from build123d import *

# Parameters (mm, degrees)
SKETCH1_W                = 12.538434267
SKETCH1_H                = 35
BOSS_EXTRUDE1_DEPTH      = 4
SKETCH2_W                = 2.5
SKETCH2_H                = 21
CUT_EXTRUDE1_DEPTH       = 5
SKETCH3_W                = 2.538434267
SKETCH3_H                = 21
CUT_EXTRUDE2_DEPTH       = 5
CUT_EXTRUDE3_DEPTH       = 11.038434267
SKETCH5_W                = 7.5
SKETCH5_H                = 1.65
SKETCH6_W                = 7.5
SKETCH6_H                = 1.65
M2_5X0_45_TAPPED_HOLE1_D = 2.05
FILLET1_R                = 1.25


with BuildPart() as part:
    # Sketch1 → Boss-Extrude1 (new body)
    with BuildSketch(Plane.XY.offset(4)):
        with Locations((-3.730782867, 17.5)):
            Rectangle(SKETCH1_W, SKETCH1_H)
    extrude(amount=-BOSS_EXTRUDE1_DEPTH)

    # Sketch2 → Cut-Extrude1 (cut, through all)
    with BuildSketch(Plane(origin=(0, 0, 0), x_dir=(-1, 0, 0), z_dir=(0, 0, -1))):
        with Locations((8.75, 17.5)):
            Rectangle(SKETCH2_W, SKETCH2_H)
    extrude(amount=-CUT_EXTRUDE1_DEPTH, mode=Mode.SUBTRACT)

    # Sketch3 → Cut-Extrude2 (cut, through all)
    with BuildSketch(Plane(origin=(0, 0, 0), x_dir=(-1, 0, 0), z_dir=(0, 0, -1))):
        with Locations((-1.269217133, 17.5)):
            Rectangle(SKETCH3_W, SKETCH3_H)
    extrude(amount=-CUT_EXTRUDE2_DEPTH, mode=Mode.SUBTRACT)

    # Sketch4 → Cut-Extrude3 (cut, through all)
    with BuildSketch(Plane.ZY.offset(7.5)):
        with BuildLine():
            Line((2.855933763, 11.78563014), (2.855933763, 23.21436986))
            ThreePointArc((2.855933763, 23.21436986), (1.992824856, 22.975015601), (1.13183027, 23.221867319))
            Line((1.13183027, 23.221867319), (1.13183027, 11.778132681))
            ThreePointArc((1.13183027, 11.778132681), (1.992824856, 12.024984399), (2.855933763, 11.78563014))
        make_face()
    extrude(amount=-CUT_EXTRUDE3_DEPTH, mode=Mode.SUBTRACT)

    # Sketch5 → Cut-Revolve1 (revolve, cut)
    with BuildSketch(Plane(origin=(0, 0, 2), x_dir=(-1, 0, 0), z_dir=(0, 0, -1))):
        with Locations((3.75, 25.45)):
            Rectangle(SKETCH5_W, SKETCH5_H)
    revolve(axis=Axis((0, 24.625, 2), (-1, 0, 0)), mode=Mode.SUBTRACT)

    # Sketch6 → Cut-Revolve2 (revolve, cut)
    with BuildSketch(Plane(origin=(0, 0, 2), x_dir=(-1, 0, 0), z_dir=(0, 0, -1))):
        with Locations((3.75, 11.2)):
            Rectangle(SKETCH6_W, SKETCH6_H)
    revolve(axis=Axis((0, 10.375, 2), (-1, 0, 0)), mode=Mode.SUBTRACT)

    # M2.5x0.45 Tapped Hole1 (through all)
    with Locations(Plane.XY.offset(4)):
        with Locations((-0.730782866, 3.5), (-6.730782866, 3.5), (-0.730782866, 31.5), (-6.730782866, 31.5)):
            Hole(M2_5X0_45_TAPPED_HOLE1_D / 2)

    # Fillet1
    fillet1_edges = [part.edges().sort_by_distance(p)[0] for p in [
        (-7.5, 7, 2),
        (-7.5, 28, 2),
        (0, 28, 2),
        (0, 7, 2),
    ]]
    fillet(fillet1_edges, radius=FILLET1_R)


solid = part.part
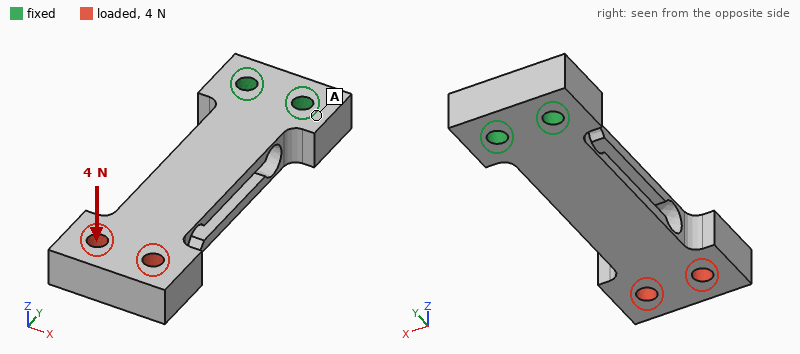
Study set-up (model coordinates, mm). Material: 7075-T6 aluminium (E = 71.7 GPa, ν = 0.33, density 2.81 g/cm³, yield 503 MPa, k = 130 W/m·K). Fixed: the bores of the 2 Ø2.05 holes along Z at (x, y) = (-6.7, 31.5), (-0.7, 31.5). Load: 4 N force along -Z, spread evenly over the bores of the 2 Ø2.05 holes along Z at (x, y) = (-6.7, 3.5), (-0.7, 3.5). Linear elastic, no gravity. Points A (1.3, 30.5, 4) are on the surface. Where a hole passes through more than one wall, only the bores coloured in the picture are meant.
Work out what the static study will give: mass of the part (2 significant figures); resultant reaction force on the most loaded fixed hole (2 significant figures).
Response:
2.8 g
2.0 N
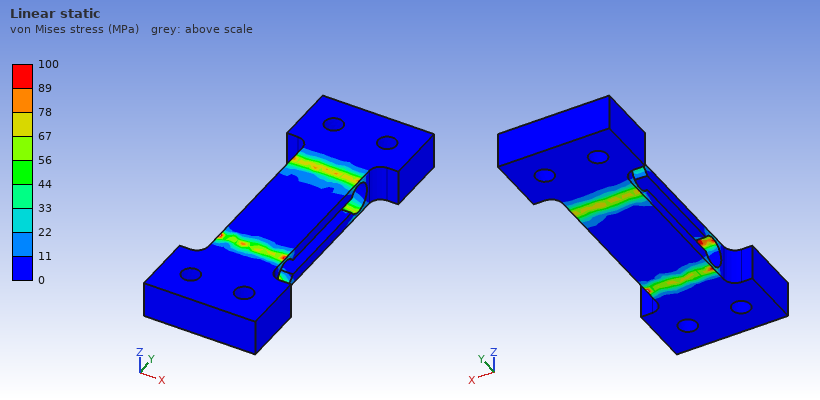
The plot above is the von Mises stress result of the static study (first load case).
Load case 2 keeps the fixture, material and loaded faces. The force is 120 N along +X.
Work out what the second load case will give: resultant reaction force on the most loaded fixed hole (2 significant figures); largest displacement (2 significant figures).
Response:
490 N
0.25 mm
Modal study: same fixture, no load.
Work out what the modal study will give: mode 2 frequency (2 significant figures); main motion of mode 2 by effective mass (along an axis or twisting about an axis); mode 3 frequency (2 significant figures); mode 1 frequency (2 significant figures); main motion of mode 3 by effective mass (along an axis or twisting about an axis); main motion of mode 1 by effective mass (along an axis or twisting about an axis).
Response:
3700 Hz
along X
4600 Hz
760 Hz
twisting about Y
along Z
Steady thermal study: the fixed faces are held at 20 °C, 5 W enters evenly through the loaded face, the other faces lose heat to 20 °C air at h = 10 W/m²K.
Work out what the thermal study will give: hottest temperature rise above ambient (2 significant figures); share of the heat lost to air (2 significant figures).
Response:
65 K
8.2 %
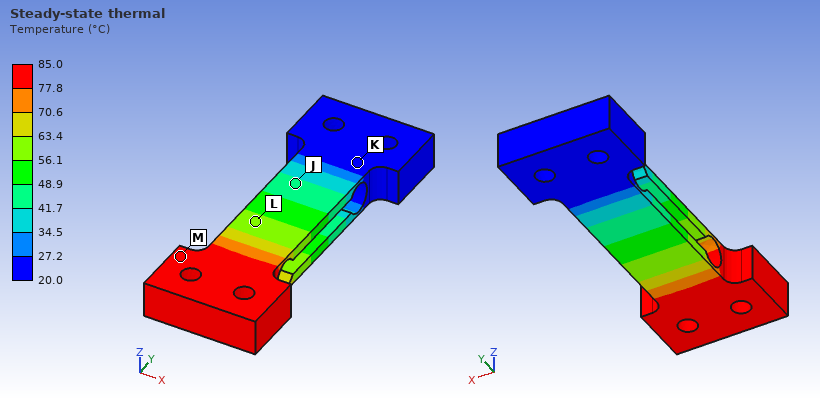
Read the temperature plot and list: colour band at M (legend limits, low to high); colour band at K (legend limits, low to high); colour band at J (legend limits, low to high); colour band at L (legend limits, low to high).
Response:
77.8 to 85.0 °C
20.0 to 27.2 °C
41.7 to 48.9 °C
56.1 to 63.4 °C
